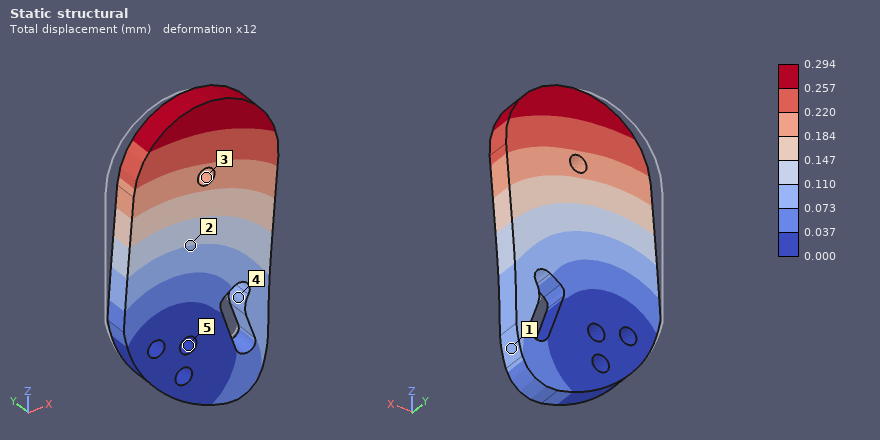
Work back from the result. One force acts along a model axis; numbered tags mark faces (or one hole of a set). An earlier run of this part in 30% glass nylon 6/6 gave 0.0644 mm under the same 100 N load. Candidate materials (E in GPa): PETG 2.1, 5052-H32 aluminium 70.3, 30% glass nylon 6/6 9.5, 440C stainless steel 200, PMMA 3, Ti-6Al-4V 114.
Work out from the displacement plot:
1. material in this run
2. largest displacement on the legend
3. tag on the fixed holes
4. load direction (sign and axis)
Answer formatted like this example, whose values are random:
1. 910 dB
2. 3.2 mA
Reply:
1. PETG
2. 0.294 mm
3. 5
4. +X
